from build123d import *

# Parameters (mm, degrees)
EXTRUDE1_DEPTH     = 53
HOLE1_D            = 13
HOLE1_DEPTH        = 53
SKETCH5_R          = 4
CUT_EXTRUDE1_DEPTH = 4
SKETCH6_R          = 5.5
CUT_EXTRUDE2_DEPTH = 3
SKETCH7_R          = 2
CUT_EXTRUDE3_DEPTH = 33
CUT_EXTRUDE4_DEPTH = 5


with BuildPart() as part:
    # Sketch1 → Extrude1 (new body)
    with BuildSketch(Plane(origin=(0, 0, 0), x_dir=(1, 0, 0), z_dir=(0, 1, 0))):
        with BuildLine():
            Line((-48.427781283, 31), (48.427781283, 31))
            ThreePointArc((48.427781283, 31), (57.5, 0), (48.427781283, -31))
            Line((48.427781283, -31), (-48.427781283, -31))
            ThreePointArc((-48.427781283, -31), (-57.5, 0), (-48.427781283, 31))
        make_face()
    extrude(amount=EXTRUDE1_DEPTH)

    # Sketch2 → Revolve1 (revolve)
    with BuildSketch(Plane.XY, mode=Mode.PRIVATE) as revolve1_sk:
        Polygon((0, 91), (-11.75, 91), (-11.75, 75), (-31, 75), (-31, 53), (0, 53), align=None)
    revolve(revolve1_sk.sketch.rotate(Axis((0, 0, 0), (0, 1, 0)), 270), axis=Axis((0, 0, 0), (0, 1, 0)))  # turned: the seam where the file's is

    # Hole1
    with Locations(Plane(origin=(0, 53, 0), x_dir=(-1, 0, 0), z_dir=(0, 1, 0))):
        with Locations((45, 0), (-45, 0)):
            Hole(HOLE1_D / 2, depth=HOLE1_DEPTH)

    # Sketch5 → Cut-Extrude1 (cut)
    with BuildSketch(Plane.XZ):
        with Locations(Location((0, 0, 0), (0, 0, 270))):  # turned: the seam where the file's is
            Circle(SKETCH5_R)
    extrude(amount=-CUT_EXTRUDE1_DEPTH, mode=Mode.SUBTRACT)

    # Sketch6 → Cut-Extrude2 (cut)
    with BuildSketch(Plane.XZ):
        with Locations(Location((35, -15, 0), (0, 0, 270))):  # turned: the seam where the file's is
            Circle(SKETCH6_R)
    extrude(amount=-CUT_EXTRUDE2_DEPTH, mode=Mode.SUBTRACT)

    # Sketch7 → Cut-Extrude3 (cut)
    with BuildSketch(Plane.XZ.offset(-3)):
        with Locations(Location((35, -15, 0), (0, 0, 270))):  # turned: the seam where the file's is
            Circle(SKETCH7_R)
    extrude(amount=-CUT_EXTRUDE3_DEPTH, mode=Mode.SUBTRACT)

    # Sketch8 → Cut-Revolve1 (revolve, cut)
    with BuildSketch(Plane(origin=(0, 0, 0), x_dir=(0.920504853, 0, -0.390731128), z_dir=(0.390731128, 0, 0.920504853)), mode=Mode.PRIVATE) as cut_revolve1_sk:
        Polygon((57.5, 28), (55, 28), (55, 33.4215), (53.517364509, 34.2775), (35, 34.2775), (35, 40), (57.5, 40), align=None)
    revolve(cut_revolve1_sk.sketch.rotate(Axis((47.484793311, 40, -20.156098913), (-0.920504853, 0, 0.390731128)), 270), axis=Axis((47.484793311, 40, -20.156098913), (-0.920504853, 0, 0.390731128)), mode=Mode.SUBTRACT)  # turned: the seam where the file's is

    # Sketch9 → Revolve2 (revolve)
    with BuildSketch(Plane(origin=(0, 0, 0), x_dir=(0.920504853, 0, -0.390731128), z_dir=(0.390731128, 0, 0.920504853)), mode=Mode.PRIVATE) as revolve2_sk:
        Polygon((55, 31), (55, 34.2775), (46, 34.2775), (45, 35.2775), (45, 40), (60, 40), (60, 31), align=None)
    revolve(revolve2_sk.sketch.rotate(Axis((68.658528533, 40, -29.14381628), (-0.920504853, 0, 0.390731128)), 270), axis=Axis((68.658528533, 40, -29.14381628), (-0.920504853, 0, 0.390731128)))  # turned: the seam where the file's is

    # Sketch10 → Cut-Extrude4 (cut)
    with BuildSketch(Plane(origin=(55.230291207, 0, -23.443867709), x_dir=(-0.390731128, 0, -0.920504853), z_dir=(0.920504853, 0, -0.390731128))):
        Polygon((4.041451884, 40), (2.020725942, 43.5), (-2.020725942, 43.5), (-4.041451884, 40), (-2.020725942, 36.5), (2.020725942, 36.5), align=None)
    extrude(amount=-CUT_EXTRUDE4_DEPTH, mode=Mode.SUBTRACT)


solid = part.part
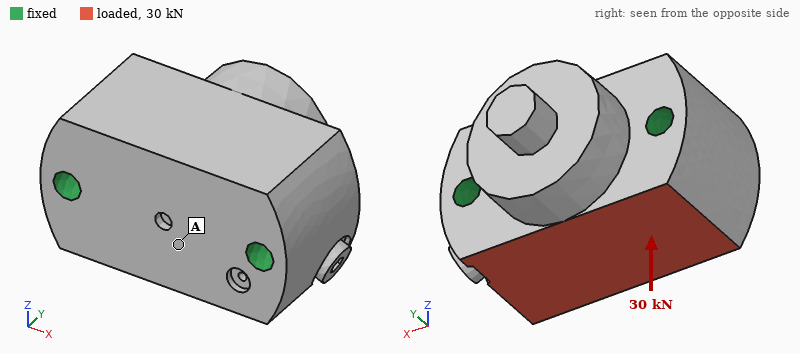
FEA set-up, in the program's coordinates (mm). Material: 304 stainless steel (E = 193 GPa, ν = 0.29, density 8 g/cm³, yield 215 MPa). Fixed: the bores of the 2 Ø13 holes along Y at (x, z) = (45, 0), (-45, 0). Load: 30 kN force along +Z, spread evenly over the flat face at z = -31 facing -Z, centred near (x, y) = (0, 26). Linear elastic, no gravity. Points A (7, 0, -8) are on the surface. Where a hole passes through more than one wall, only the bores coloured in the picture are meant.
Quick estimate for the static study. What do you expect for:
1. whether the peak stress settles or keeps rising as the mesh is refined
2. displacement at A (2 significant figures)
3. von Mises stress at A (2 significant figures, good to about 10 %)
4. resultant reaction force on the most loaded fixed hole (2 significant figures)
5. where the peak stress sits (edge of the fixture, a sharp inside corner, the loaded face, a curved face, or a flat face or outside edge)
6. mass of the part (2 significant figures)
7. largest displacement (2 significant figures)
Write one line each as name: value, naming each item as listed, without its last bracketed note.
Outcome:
whether the peak stress settles or keeps rising as the mesh is refined: keeps rising
displacement at A: 2.4 µm
von Mises stress at A: 4.1 MPa
resultant reaction force on the most loaded fixed hole: 15 kN
where the peak stress sits: a sharp inside corner
mass of the part: 3.3 kg
largest displacement: 2.9 µm
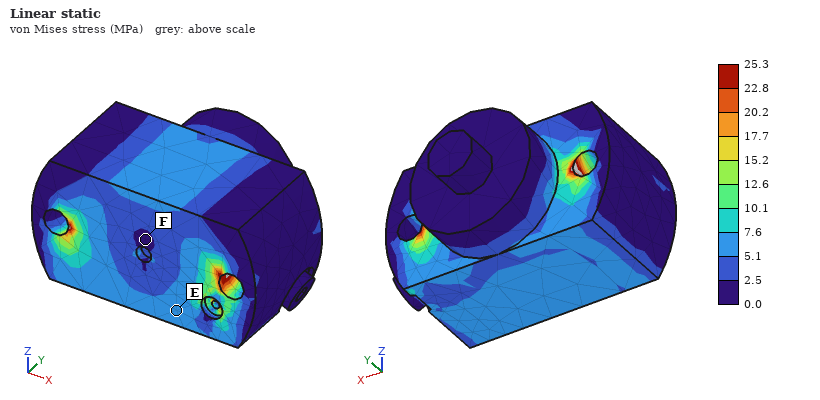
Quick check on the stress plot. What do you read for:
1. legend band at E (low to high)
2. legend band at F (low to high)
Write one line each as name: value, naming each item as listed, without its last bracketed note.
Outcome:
legend band at E: 5.1 to 7.6 MPa
legend band at F: 0.0 to 2.5 MPa
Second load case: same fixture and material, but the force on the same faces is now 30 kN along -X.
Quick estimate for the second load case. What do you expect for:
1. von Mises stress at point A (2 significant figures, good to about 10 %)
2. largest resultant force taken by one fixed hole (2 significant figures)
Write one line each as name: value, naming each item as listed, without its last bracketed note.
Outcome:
von Mises stress at point A: 6.8 MPa
largest resultant force taken by one fixed hole: 18 kN
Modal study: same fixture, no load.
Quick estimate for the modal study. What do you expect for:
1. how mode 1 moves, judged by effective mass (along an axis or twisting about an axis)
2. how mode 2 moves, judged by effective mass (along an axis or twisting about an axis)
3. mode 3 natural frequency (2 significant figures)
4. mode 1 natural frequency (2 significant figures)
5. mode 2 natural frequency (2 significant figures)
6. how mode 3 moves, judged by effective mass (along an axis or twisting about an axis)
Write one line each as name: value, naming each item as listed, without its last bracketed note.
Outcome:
how mode 1 moves, judged by effective mass: along Z
how mode 2 moves, judged by effective mass: along Y
mode 3 natural frequency: 13 kHz
mode 1 natural frequency: 8000 Hz
mode 2 natural frequency: 11 kHz
how mode 3 moves, judged by effective mass: along Z
